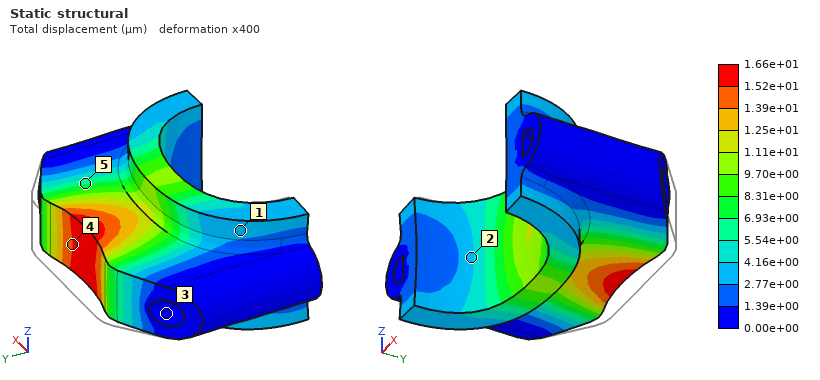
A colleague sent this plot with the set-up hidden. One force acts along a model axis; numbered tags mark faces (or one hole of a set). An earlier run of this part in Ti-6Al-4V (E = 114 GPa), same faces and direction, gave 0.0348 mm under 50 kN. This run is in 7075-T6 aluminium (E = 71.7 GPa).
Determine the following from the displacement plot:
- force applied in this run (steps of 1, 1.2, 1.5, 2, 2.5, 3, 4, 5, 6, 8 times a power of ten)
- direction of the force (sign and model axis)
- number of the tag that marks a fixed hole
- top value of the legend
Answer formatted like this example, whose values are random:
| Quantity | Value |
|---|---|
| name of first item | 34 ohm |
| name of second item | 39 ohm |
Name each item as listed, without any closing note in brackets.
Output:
| Quantity | Value |
|---|---|
| force applied in this run | 15 kN |
| direction of the force | -Y |
| number of the tag that marks a fixed hole | 3 |
| top value of the legend | 1.66e+01 µm |
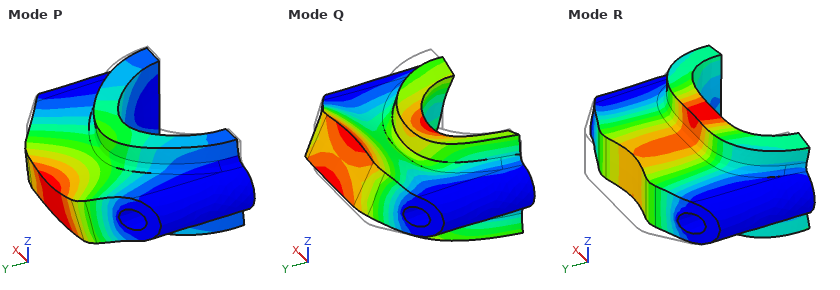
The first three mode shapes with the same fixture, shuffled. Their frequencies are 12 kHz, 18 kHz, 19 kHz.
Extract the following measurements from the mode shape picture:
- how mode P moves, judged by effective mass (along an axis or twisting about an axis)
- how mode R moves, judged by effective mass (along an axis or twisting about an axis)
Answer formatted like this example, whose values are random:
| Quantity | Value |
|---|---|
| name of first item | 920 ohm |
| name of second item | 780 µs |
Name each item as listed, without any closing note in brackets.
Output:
| Quantity | Value |
|---|---|
| how mode P moves, judged by effective mass | along Z |
| how mode R moves, judged by effective mass | along Y |
